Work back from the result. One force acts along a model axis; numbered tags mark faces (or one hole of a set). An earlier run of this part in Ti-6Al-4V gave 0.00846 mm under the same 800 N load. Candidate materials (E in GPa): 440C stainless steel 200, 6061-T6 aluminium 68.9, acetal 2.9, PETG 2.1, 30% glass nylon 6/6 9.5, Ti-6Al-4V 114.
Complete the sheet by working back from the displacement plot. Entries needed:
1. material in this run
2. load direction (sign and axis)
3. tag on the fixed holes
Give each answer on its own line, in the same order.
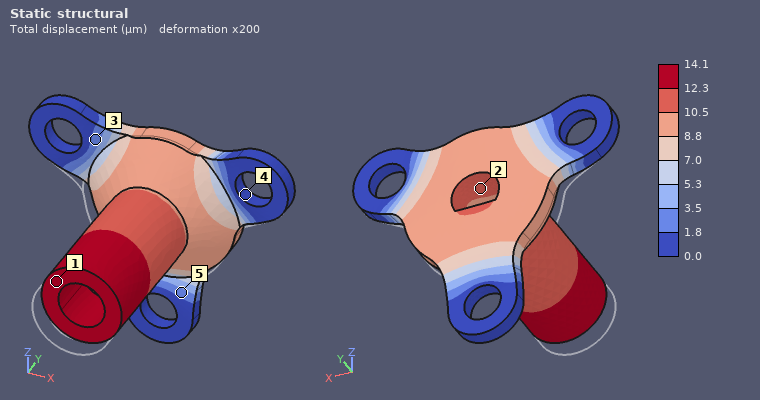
6061-T6 aluminium
+Y
4
